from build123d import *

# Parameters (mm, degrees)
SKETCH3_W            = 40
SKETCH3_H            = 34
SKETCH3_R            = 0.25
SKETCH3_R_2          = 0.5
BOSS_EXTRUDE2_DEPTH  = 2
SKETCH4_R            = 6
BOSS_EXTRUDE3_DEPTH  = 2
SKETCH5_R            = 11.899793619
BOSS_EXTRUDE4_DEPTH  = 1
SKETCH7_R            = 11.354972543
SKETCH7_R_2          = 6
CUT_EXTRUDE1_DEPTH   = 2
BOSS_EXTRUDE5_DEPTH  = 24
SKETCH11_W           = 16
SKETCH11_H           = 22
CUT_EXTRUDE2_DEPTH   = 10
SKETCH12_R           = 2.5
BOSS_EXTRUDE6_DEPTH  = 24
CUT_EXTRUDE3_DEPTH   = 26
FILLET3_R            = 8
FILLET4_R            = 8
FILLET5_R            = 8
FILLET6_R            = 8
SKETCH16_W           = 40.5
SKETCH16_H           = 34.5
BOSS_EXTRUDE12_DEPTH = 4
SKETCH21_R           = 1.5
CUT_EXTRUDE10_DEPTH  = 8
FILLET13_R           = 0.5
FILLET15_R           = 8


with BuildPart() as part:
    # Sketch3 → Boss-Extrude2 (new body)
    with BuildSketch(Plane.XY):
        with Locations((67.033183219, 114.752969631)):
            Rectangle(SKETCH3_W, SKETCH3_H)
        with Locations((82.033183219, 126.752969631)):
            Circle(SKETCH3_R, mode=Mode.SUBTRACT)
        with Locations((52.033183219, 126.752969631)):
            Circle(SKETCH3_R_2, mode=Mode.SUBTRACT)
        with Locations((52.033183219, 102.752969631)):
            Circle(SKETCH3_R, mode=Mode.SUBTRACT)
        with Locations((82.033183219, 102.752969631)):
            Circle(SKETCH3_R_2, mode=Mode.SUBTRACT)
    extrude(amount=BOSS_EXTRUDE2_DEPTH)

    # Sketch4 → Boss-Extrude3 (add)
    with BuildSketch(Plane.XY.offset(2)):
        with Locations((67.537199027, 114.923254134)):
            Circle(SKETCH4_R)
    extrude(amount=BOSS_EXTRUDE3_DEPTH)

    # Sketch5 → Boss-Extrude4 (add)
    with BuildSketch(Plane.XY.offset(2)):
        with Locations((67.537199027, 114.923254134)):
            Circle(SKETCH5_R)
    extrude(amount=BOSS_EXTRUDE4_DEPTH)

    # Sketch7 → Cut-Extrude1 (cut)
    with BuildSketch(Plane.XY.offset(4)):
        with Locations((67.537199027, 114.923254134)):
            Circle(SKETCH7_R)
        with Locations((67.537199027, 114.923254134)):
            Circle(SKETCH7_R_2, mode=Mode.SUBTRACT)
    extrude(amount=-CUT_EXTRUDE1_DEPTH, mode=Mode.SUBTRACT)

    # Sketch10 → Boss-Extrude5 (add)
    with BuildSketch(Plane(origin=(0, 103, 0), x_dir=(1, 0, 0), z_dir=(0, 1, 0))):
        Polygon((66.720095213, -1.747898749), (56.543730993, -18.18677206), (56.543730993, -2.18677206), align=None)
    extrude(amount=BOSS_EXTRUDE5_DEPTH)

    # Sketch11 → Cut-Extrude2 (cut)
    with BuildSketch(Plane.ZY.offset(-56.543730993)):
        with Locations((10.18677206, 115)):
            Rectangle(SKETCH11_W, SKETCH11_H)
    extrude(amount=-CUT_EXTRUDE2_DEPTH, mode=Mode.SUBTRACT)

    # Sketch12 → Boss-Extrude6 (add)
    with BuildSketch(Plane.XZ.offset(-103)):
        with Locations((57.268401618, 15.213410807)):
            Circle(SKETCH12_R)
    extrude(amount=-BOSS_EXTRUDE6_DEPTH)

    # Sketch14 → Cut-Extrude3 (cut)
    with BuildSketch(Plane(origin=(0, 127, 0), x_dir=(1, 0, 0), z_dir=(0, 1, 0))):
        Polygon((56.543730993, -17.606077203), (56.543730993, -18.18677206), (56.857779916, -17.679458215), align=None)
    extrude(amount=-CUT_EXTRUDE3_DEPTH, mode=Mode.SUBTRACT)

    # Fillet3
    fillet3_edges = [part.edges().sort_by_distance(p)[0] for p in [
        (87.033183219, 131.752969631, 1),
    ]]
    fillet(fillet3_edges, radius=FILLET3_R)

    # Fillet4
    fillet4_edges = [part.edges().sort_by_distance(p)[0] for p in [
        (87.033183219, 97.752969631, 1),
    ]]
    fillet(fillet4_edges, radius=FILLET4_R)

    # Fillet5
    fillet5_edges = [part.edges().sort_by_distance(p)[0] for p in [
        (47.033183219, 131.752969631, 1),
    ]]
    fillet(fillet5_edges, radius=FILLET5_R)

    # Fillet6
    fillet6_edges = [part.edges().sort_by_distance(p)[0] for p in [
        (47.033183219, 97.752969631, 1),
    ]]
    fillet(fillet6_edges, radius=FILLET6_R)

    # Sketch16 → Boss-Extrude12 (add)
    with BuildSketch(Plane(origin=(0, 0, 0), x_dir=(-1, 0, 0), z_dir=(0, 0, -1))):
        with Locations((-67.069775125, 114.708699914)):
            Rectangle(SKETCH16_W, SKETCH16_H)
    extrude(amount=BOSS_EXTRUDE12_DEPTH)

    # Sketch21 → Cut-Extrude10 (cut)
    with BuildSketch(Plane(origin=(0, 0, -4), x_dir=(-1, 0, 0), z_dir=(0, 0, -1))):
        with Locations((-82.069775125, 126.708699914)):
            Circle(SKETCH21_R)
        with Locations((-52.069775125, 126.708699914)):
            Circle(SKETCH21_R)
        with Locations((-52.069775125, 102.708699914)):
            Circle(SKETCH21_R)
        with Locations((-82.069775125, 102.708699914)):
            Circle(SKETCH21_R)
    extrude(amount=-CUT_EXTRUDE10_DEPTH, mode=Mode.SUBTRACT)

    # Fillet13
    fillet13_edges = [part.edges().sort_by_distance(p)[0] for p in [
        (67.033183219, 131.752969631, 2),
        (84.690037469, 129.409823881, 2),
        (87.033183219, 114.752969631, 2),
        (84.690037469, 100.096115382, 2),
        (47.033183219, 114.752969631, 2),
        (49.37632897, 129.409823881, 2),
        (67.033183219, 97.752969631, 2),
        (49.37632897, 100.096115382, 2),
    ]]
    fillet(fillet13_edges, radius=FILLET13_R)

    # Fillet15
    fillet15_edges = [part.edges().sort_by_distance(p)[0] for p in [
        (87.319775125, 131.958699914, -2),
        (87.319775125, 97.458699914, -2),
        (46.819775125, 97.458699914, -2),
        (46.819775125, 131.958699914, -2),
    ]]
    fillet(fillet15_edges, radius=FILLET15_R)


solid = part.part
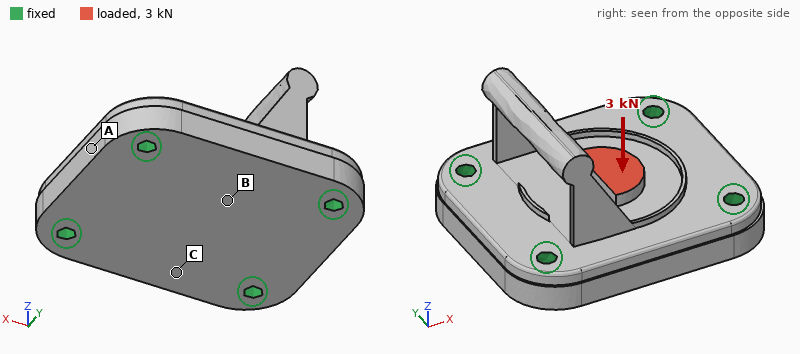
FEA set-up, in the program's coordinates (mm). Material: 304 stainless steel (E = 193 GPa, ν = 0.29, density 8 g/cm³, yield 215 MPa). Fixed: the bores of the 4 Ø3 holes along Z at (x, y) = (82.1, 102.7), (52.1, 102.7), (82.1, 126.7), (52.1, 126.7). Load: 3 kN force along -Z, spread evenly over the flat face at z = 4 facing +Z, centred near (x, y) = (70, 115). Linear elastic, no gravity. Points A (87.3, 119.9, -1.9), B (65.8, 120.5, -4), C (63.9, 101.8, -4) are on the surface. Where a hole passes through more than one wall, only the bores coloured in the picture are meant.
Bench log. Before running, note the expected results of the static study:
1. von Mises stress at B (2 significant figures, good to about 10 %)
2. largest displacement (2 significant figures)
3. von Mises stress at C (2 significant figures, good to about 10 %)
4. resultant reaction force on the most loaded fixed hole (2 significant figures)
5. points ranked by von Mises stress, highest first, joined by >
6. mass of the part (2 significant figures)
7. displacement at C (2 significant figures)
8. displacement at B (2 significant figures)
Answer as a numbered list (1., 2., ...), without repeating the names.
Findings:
1. 44 MPa
2. 8.8 µm
3. 25 MPa
4. 920 N
5. B > C > A
6. 69 g
7. 3.6 µm
8. 6.7 µm
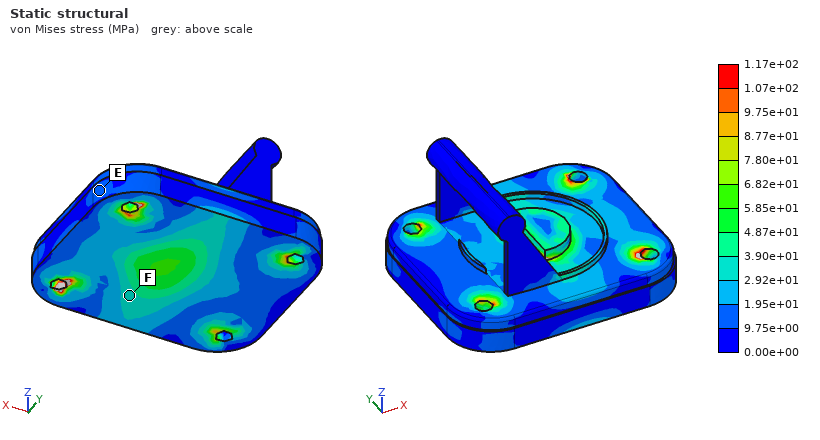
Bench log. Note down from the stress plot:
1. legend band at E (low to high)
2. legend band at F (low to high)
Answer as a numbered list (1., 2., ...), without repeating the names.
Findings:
1. 9.75e+00 to 1.95e+01 MPa
2. 2.92e+01 to 3.90e+01 MPa
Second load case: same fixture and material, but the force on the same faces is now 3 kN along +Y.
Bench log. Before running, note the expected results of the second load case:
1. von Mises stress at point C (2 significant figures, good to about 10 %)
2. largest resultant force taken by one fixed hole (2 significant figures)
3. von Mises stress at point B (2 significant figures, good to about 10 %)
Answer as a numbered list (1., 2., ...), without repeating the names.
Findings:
1. 15 MPa
2. 1.0 kN
3. 18 MPa
